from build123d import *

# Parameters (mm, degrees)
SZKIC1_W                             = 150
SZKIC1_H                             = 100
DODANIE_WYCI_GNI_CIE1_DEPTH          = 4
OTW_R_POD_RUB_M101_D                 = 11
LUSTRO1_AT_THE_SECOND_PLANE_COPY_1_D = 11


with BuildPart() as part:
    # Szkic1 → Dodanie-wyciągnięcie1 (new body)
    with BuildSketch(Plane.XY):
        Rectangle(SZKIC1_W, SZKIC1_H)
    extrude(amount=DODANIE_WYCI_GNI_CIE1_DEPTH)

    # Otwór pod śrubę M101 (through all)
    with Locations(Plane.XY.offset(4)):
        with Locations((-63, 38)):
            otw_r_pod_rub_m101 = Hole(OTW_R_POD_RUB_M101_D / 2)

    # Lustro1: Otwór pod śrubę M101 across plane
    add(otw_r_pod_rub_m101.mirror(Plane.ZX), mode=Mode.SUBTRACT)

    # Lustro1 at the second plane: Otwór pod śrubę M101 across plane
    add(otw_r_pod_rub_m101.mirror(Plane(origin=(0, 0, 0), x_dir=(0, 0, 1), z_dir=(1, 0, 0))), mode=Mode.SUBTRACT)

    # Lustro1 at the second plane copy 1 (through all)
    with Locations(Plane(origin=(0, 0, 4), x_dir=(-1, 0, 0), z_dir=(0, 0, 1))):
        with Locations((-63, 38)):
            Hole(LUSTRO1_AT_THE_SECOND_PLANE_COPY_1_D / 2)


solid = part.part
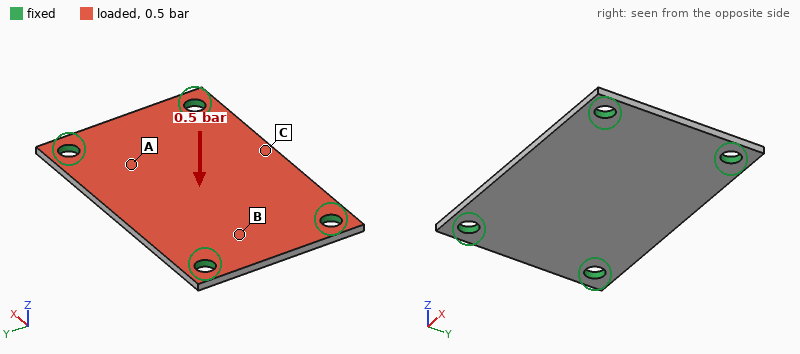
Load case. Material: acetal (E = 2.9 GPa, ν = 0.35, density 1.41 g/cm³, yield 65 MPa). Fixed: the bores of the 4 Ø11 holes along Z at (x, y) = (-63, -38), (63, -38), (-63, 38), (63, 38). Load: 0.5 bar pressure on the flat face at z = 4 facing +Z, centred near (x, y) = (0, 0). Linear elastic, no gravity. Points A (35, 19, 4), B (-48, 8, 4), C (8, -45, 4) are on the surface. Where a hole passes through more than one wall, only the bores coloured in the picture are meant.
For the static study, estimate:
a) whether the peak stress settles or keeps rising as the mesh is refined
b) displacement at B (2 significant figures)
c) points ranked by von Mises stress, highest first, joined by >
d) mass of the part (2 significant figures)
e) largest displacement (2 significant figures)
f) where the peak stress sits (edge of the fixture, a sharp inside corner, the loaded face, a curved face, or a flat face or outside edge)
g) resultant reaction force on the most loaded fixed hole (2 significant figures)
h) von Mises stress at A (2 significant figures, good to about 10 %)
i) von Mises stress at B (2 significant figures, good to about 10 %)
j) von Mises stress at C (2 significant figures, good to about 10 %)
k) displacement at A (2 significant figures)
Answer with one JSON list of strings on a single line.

["keeps rising", "0.70 mm", "C > B > A", "82 g", "2.1 mm", "edge of the fixture", "180 N", "3.4 MPa", "6.4 MPa", "12 MPa", "1.1 mm"]
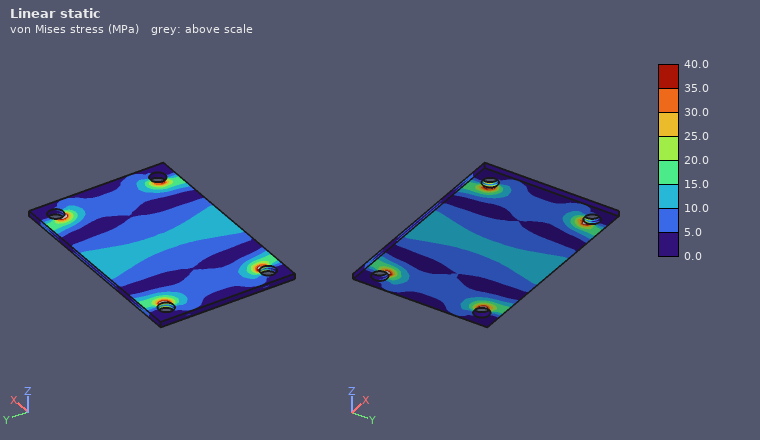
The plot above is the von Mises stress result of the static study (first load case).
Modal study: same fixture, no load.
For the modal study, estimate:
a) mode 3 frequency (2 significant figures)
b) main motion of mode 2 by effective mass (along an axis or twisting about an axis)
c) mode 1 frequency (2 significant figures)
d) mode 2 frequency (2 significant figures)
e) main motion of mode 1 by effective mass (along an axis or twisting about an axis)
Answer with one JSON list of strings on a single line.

["900 Hz", "twisting about X", "370 Hz", "530 Hz", "along Z"]
